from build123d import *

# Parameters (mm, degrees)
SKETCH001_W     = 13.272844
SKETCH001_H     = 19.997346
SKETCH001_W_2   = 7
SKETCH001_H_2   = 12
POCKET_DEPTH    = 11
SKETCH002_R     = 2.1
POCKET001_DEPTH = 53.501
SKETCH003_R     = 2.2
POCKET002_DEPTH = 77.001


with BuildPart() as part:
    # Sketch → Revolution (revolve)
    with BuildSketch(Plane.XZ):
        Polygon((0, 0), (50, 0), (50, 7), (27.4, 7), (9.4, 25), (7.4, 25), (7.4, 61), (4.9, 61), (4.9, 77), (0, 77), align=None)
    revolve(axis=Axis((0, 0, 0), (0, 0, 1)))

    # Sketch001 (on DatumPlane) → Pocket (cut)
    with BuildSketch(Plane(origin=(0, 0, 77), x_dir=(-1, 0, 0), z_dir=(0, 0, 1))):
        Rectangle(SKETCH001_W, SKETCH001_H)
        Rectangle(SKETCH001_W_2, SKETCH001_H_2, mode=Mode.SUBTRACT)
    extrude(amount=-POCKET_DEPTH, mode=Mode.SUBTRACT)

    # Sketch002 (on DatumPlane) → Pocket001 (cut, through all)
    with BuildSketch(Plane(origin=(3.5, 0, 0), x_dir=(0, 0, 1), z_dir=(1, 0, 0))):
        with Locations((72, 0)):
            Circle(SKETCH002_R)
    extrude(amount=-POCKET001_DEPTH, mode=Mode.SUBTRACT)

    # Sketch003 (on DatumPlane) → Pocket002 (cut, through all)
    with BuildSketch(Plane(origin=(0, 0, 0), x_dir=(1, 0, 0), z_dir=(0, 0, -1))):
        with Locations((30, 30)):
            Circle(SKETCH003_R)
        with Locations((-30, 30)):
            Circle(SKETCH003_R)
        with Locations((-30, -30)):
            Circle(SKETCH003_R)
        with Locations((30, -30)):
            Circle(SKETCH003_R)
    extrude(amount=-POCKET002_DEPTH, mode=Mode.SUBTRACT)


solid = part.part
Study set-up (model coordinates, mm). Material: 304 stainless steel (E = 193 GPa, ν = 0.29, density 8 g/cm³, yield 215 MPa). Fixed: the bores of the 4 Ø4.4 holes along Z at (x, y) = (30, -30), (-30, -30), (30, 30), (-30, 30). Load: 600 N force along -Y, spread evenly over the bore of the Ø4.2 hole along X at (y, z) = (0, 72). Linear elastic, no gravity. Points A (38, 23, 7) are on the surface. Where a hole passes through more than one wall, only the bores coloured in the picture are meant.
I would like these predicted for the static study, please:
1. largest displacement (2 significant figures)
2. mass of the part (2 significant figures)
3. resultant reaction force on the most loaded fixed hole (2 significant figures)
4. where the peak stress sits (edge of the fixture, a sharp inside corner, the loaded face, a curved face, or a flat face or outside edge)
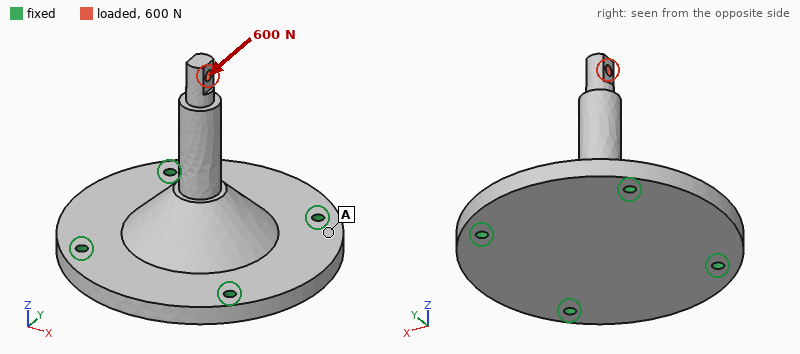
83 µm
660 g
410 N
a curved face
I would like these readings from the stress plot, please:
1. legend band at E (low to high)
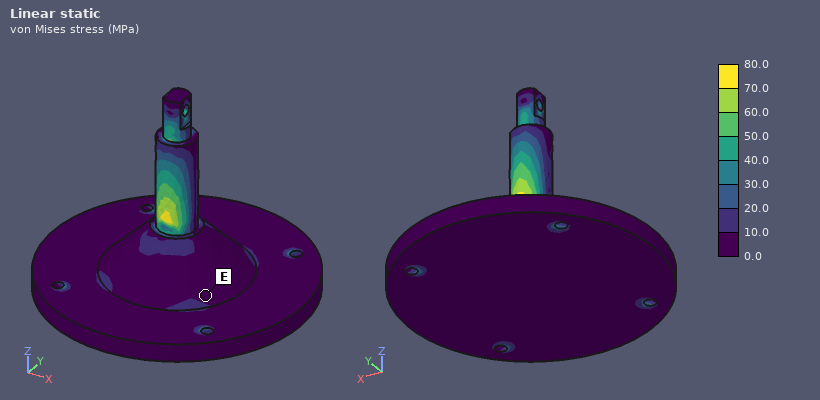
0.0 to 10.0 MPa
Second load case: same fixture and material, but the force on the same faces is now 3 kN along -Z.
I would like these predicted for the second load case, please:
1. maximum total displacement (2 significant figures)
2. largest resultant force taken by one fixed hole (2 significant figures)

14 µm
820 N
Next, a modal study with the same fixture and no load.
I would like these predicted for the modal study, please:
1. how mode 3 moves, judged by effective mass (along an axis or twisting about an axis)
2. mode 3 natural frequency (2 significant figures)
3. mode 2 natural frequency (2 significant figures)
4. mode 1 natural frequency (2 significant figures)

along Z
5700 Hz
4000 Hz
4000 Hz
